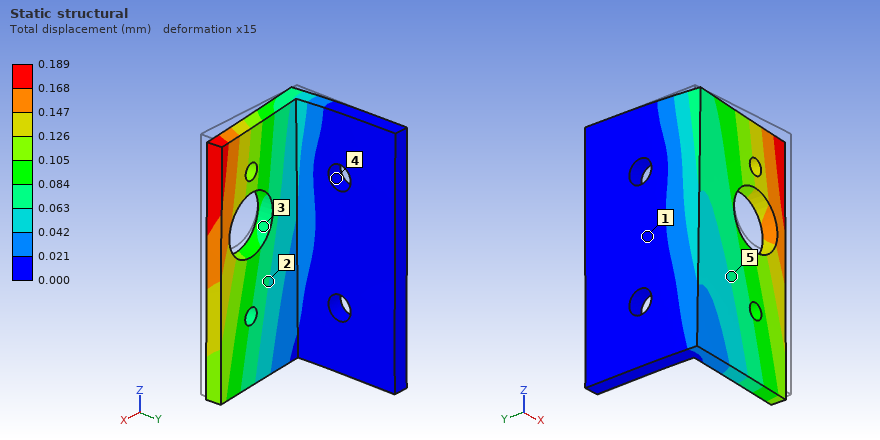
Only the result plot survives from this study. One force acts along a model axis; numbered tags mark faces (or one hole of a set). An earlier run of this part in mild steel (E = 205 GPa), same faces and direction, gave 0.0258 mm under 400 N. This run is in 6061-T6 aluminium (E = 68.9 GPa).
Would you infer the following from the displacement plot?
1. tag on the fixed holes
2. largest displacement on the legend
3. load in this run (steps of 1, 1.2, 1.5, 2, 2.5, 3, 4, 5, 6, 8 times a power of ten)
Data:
4
0.189 mm
1 kN
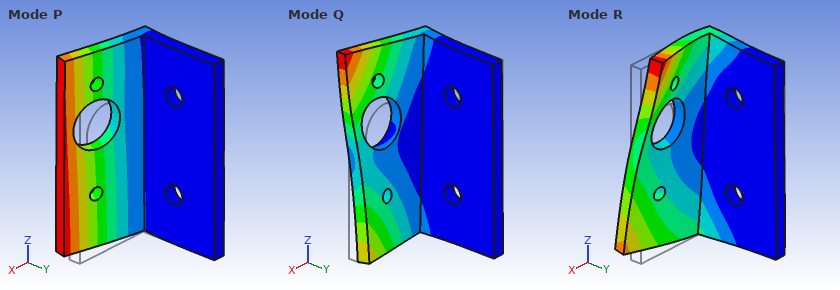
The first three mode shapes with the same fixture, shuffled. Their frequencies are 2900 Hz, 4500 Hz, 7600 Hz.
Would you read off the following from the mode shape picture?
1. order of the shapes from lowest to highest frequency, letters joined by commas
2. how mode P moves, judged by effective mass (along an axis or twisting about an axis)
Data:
P, Q, R
along Y
